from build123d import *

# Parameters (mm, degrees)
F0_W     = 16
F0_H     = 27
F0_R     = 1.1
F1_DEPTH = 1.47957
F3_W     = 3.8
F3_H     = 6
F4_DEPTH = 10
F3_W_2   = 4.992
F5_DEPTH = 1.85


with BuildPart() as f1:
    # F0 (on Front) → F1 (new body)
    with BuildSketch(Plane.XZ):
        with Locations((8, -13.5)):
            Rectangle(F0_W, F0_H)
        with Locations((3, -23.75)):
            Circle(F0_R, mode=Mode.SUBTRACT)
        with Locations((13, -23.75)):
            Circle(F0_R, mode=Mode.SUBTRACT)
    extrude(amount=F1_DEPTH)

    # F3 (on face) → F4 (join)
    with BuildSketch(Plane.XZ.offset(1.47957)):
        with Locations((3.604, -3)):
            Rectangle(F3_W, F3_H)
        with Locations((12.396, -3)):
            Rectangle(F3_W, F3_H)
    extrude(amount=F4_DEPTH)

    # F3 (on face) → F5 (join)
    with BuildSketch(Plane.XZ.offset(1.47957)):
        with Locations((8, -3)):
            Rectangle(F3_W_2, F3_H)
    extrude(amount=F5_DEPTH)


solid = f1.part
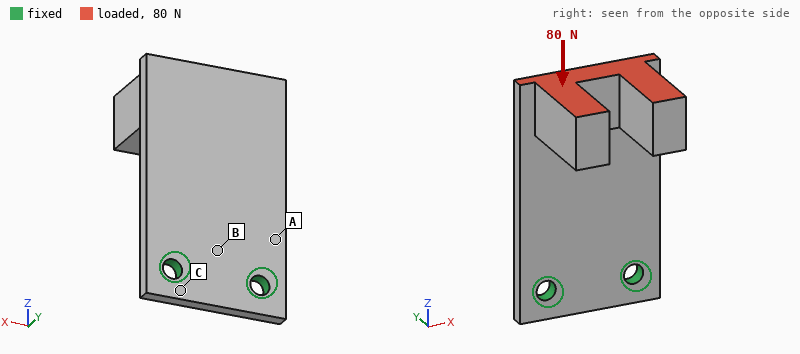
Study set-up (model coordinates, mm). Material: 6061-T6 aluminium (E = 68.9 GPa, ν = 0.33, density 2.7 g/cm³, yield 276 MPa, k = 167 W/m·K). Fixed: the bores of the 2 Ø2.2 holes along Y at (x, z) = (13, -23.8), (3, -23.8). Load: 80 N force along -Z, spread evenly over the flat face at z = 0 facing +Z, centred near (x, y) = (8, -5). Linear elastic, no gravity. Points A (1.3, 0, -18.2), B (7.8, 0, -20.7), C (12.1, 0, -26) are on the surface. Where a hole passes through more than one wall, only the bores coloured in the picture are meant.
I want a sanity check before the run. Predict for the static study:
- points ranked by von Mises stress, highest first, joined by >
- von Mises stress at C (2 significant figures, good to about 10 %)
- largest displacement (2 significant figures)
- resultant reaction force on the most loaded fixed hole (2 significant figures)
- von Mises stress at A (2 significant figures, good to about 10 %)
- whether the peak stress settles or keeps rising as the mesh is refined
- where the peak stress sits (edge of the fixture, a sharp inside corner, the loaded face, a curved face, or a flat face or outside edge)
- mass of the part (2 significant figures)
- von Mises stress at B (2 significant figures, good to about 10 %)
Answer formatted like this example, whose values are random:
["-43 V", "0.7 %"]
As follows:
["A > B > C", "8.5 MPa", "0.35 mm", "40 N", "55 MPa", "keeps rising", "edge of the fixture", "3.1 g", "45 MPa"]
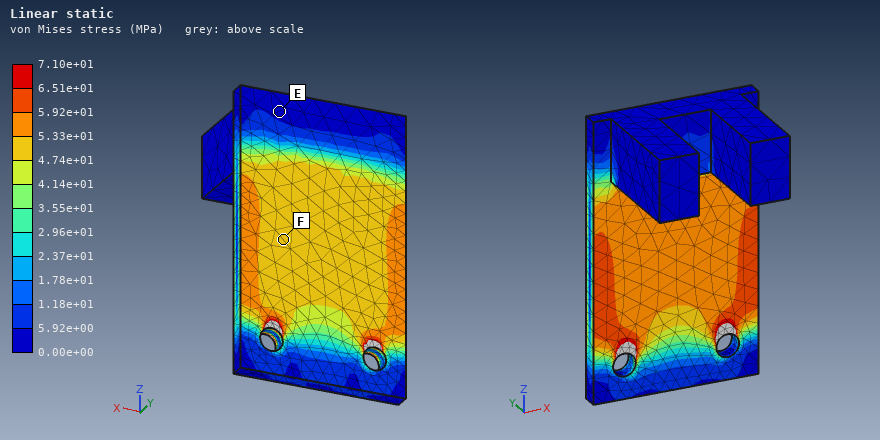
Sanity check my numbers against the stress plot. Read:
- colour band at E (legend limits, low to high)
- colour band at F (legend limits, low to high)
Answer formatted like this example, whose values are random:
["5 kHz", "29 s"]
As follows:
["0.00e+00 to 5.92e+00 MPa", "4.74e+01 to 5.33e+01 MPa"]
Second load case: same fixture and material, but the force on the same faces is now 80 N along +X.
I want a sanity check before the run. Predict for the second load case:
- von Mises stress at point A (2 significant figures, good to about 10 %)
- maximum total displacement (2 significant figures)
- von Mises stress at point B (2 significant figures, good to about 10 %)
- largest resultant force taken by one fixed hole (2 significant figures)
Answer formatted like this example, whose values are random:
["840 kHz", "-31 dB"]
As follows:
["47 MPa", "0.12 mm", "15 MPa", "180 N"]
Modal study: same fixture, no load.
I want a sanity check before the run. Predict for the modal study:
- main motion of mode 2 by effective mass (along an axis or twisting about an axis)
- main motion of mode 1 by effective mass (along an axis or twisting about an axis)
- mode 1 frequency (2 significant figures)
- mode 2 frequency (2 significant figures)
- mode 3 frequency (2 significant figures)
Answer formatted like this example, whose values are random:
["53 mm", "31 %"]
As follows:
["along X", "along Y", "1100 Hz", "3100 Hz", "6100 Hz"]
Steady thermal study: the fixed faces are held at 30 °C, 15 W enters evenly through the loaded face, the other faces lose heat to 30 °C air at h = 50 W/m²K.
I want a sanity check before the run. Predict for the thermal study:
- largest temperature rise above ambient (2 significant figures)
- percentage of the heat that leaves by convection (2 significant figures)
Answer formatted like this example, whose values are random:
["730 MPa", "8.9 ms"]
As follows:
["71 K", "17 %"]
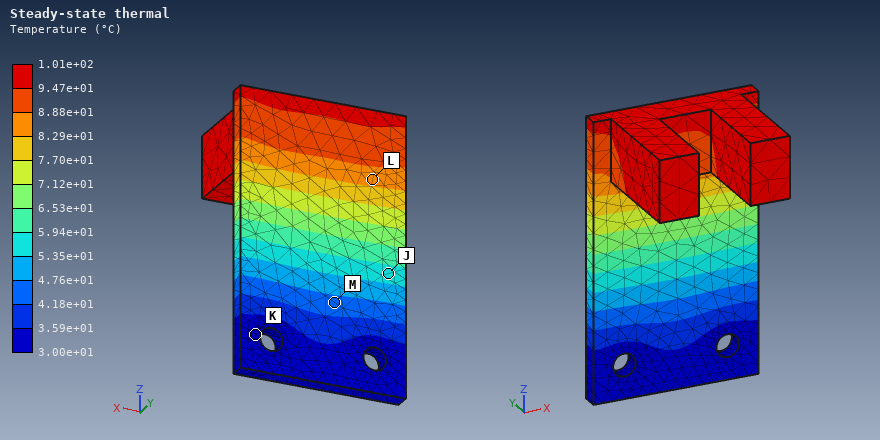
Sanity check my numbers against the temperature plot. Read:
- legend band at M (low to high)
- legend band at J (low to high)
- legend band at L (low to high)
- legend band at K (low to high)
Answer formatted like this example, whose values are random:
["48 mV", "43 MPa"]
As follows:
["4.18e+01 to 4.76e+01 °C", "5.35e+01 to 5.94e+01 °C", "8.29e+01 to 8.88e+01 °C", "3.00e+01 to 3.59e+01 °C"]
